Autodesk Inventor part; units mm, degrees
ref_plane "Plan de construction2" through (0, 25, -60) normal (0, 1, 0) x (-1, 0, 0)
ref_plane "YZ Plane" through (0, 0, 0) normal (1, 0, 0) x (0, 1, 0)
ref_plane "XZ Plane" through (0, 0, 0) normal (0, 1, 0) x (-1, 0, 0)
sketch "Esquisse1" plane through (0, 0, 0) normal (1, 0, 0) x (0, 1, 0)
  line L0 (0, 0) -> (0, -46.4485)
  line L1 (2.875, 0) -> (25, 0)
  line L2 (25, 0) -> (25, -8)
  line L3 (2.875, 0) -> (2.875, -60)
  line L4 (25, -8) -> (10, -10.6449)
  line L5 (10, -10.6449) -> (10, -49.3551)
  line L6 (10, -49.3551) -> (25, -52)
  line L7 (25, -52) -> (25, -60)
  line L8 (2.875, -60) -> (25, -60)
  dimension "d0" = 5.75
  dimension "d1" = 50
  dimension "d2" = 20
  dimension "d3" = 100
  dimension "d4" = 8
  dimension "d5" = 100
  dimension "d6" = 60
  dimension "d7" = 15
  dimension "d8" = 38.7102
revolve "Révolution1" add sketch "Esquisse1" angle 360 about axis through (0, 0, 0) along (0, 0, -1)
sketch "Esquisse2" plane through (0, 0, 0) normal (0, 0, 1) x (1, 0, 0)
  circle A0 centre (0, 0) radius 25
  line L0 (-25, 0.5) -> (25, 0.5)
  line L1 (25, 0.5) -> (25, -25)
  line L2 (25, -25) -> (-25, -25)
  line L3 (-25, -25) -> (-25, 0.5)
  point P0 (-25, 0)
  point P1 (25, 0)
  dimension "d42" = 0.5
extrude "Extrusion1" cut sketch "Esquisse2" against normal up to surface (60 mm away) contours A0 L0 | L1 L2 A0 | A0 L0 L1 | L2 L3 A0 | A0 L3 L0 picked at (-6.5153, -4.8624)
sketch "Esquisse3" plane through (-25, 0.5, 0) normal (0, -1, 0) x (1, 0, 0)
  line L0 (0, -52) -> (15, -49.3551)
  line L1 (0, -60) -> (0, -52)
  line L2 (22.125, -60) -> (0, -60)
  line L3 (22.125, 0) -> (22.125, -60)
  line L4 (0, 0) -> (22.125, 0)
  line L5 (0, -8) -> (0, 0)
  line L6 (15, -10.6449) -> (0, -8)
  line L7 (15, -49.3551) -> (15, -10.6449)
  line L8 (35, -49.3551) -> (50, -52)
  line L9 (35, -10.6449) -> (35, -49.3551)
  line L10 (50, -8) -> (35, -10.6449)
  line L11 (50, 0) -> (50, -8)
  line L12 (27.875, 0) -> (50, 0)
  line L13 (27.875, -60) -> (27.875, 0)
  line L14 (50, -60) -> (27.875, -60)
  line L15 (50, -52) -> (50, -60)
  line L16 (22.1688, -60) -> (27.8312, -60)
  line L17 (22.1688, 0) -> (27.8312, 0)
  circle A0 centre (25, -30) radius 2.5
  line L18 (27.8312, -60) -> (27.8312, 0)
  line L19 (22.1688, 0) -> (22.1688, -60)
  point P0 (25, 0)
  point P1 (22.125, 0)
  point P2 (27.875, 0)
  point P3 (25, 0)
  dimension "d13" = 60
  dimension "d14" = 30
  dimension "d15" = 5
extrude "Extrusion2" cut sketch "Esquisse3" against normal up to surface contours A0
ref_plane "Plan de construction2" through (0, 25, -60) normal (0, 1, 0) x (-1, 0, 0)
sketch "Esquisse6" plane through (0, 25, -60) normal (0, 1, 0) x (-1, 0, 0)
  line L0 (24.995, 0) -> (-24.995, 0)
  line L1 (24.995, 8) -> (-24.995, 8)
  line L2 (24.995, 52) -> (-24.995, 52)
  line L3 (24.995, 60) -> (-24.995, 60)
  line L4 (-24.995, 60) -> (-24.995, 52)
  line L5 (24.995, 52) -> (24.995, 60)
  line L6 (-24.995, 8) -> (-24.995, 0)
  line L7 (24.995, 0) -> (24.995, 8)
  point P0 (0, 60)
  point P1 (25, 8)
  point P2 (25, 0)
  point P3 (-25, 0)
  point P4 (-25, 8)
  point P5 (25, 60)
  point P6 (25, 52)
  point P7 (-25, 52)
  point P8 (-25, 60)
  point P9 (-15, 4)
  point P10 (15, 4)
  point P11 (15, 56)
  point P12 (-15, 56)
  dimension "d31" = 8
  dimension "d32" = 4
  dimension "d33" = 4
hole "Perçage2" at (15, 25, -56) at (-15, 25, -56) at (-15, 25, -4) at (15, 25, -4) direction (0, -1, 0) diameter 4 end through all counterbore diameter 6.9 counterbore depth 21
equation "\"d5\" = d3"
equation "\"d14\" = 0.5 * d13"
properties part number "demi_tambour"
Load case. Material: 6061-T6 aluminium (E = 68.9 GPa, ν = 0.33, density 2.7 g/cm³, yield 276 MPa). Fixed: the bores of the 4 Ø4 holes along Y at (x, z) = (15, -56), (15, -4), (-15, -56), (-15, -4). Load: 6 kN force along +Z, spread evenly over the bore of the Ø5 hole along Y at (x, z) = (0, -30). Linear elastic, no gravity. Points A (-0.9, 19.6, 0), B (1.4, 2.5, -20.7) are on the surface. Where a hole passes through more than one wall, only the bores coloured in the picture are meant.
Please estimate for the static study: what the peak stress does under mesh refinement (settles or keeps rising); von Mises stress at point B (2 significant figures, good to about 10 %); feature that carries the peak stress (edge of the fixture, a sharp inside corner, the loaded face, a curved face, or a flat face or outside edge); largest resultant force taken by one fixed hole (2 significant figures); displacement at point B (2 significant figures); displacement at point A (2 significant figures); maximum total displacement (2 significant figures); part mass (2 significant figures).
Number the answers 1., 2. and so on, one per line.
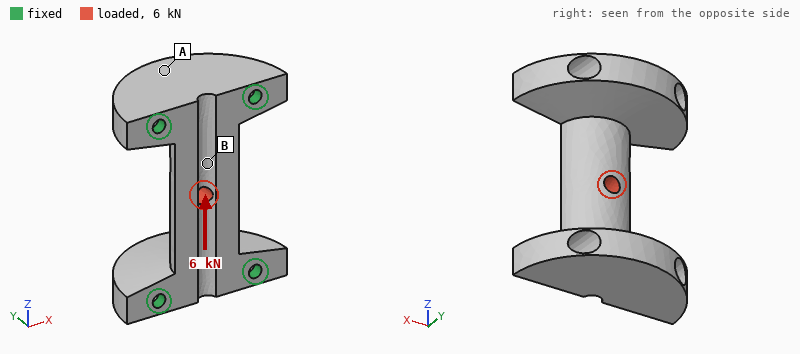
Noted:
1. keeps rising
2. 30 MPa
3. edge of the fixture
4. 1.6 kN
5. 16 µm
6. 17 µm
7. 21 µm
8. 55 g
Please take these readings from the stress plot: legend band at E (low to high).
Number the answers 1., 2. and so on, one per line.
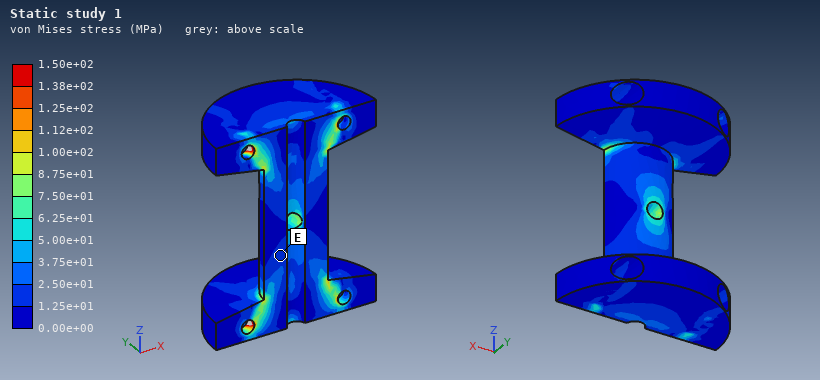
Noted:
1. 1.25e+01 to 2.50e+01 MPa
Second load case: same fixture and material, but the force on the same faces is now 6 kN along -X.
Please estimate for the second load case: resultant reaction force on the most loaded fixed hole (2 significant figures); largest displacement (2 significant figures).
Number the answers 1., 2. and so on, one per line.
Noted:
1. 2.1 kN
2. 46 µm
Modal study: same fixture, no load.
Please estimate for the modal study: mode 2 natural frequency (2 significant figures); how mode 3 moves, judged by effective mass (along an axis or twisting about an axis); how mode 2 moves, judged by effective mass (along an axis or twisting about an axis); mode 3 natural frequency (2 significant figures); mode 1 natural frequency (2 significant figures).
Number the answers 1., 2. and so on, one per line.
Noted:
1. 10 kHz
2. along Y
3. along Z
4. 18 kHz
5. 7500 Hz
